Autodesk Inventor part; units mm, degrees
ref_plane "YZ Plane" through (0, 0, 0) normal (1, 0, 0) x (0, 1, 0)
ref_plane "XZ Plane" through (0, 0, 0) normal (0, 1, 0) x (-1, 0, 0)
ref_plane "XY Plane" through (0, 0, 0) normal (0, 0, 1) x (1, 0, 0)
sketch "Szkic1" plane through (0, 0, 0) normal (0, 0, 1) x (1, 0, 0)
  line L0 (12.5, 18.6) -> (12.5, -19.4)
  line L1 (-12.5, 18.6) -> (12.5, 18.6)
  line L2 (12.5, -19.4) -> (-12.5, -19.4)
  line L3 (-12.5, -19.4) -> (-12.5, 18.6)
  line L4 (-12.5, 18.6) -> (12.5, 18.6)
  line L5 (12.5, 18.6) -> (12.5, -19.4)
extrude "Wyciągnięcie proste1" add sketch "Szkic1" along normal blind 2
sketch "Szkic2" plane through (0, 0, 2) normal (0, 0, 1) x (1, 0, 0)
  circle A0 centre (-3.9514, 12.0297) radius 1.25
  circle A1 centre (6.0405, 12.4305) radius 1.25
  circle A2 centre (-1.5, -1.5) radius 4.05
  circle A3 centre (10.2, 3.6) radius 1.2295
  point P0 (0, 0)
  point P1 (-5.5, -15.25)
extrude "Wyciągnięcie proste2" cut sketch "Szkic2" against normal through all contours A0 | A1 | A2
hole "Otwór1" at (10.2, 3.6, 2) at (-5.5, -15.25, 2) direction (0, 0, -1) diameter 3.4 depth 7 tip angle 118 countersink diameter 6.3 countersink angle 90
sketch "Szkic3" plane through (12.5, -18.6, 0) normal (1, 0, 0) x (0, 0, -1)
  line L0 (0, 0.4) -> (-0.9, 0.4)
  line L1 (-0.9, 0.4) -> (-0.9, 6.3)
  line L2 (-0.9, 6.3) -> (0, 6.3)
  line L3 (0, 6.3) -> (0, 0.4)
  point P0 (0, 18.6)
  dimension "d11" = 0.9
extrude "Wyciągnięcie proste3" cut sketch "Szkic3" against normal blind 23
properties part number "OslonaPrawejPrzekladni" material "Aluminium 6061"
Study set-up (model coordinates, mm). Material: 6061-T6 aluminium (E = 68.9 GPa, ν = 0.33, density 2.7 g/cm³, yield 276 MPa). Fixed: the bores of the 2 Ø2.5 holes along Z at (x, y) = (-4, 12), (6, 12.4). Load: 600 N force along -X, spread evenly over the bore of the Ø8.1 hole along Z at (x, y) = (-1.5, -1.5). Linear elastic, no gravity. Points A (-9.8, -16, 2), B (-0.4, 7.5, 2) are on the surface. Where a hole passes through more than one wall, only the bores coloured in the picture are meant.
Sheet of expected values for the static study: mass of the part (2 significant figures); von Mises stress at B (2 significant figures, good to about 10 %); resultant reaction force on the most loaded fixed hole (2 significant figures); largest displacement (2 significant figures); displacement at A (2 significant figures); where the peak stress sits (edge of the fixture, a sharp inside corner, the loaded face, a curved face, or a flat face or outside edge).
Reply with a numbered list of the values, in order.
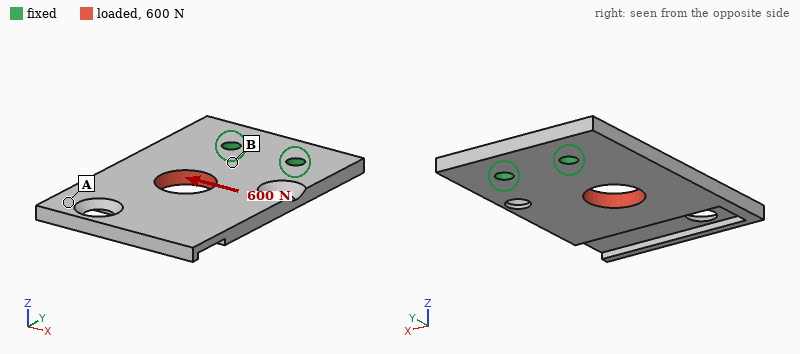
1. 4.3 g
2. 54 MPa
3. 760 N
4. 44 µm
5. 39 µm
6. a curved face
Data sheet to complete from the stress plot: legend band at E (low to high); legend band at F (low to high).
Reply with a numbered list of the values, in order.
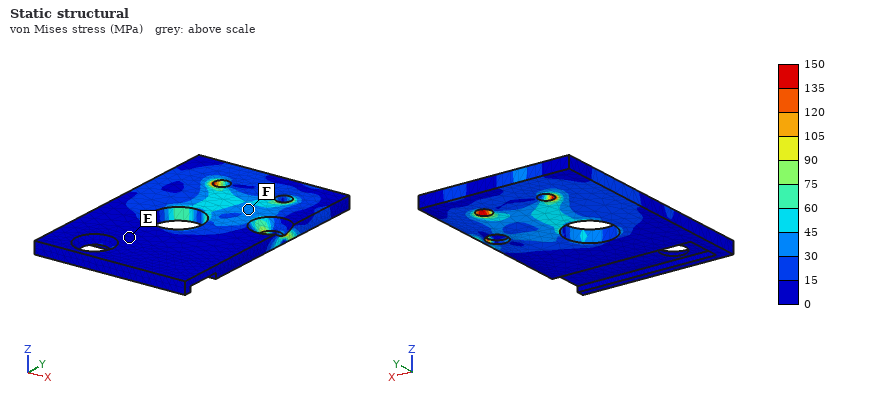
1. 0 to 15 MPa
2. 30 to 45 MPa
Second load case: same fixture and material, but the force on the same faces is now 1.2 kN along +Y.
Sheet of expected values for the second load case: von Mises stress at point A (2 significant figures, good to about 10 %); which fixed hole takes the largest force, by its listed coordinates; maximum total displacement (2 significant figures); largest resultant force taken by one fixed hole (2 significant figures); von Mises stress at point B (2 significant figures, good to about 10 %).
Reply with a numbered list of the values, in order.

1. 9.5 MPa
2. (-4, 12)
3. 16 µm
4. 860 N
5. 31 MPa
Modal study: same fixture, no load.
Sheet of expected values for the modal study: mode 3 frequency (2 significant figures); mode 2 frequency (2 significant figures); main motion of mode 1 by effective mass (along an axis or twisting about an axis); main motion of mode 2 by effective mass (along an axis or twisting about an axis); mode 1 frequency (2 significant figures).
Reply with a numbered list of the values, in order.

1. 9500 Hz
2. 4200 Hz
3. along Z
4. twisting about Y
5. 1700 Hz
